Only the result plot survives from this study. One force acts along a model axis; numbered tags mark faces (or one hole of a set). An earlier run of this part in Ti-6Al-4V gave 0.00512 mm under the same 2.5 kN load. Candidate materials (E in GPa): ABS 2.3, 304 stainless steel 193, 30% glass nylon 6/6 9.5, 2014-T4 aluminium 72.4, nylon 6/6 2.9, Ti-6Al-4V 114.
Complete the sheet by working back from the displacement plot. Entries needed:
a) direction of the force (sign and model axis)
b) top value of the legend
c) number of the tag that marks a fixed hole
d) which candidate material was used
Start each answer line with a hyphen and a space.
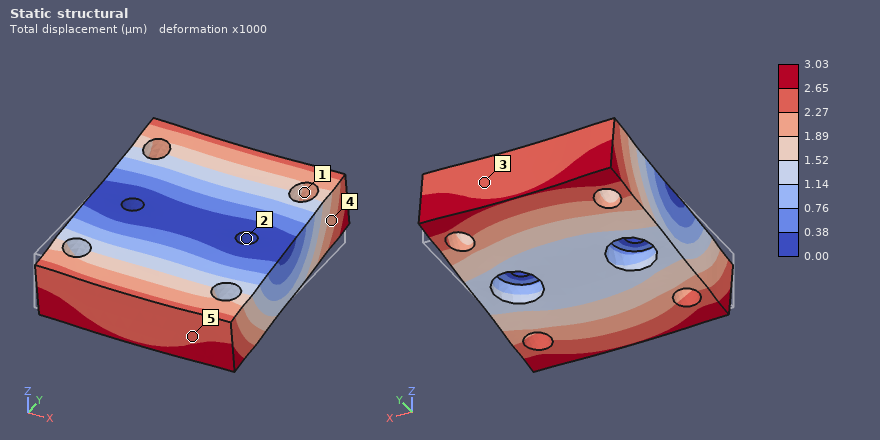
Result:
- +Y
- 3.03 µm
- 2
- 304 stainless steel
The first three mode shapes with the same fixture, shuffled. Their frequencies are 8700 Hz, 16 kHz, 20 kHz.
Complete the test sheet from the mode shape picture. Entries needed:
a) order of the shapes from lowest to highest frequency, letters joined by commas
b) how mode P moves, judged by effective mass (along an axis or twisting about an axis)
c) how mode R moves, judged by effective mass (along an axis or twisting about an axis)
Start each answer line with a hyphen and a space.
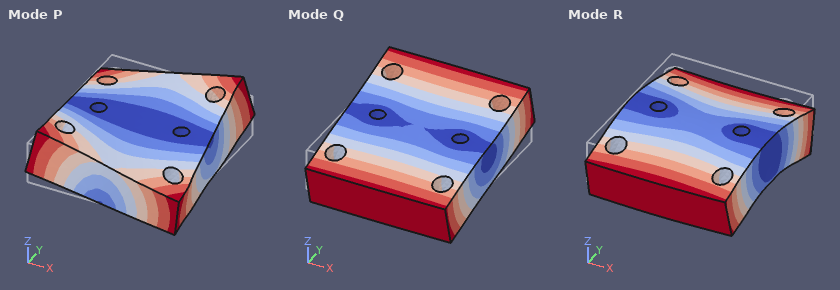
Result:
- Q, R, P
- twisting about Z
- along Z
